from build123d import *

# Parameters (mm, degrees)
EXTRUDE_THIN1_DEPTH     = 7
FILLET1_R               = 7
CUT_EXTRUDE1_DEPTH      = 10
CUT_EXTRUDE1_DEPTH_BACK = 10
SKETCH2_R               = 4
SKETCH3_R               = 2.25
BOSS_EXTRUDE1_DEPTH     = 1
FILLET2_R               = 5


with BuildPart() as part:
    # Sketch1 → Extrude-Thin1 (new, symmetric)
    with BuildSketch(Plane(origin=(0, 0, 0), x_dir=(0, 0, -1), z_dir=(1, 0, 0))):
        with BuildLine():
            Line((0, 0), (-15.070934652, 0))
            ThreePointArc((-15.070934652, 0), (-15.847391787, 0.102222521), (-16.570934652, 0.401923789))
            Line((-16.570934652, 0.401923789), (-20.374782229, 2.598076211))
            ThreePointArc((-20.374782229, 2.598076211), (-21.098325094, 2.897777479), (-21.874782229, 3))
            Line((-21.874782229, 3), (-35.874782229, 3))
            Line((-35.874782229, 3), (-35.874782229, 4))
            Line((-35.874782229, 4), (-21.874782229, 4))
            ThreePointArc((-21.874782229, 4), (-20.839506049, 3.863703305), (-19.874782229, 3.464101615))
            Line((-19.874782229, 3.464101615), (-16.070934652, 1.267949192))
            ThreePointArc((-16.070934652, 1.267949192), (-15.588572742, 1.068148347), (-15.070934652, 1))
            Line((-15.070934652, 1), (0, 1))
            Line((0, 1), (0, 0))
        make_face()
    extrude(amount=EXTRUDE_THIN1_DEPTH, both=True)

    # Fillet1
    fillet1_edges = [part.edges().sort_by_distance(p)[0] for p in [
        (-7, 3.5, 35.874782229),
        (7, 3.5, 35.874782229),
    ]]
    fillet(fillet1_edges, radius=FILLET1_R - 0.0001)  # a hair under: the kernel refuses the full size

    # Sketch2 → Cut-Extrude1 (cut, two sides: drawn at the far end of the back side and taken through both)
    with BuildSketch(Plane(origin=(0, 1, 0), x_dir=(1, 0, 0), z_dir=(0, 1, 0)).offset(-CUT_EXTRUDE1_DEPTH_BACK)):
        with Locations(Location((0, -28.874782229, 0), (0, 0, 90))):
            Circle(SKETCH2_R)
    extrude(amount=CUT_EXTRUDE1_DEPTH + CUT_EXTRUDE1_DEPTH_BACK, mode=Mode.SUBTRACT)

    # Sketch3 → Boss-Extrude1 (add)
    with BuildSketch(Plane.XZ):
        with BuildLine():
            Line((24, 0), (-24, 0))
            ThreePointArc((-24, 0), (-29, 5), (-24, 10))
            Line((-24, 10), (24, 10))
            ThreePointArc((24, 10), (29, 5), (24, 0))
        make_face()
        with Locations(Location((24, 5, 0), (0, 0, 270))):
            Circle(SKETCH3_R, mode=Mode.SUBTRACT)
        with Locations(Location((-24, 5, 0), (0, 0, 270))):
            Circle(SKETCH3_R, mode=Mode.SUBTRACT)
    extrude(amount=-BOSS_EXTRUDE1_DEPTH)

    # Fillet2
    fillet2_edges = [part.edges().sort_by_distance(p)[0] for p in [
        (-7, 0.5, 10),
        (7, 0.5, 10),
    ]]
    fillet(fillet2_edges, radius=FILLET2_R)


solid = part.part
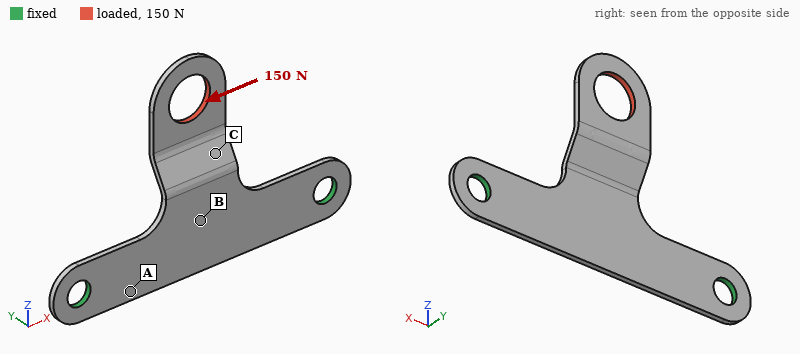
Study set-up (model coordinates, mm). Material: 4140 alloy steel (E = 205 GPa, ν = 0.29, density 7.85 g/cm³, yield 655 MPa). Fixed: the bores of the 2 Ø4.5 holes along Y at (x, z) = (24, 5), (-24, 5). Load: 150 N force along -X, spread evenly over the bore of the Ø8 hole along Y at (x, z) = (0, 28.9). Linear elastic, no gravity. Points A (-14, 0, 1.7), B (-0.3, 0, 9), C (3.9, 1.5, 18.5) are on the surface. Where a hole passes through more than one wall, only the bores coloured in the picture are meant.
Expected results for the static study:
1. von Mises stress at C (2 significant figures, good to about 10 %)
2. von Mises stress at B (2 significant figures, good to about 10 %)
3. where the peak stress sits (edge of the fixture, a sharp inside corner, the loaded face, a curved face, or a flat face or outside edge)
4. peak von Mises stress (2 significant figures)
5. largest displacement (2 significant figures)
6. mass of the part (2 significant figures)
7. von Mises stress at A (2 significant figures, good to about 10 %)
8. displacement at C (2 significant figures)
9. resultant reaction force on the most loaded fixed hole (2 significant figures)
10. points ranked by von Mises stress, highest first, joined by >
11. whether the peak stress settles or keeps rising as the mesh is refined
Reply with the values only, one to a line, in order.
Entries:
120 MPa
80 MPa
a curved face
360 MPa
75 µm
6.6 g
33 MPa
23 µm
120 N
C > B > A
settles
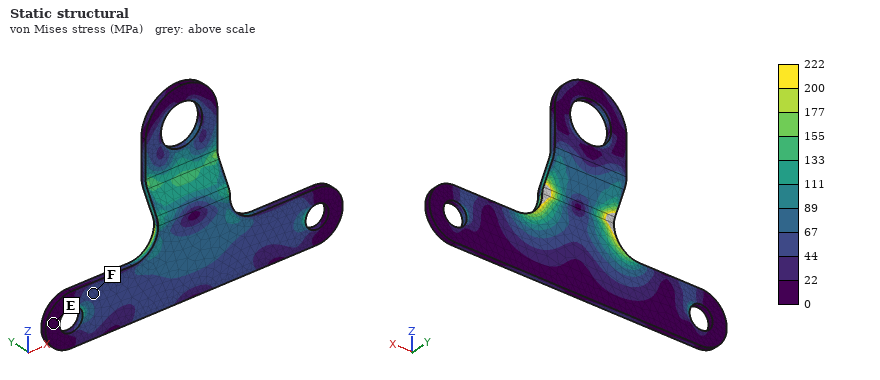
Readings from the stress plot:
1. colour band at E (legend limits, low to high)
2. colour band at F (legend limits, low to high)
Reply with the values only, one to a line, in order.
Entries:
0 to 22 MPa
44 to 67 MPa
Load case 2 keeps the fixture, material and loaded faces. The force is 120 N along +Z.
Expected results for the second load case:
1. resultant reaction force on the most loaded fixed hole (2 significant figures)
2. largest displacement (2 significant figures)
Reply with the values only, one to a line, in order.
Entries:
65 N
0.66 mm
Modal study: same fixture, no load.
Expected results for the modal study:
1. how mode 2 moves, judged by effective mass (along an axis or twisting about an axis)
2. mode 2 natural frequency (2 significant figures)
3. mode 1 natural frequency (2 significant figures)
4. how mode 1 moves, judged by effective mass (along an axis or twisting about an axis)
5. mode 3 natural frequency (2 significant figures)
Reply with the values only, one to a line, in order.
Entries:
along Y
2500 Hz
830 Hz
along Y
4200 Hz
